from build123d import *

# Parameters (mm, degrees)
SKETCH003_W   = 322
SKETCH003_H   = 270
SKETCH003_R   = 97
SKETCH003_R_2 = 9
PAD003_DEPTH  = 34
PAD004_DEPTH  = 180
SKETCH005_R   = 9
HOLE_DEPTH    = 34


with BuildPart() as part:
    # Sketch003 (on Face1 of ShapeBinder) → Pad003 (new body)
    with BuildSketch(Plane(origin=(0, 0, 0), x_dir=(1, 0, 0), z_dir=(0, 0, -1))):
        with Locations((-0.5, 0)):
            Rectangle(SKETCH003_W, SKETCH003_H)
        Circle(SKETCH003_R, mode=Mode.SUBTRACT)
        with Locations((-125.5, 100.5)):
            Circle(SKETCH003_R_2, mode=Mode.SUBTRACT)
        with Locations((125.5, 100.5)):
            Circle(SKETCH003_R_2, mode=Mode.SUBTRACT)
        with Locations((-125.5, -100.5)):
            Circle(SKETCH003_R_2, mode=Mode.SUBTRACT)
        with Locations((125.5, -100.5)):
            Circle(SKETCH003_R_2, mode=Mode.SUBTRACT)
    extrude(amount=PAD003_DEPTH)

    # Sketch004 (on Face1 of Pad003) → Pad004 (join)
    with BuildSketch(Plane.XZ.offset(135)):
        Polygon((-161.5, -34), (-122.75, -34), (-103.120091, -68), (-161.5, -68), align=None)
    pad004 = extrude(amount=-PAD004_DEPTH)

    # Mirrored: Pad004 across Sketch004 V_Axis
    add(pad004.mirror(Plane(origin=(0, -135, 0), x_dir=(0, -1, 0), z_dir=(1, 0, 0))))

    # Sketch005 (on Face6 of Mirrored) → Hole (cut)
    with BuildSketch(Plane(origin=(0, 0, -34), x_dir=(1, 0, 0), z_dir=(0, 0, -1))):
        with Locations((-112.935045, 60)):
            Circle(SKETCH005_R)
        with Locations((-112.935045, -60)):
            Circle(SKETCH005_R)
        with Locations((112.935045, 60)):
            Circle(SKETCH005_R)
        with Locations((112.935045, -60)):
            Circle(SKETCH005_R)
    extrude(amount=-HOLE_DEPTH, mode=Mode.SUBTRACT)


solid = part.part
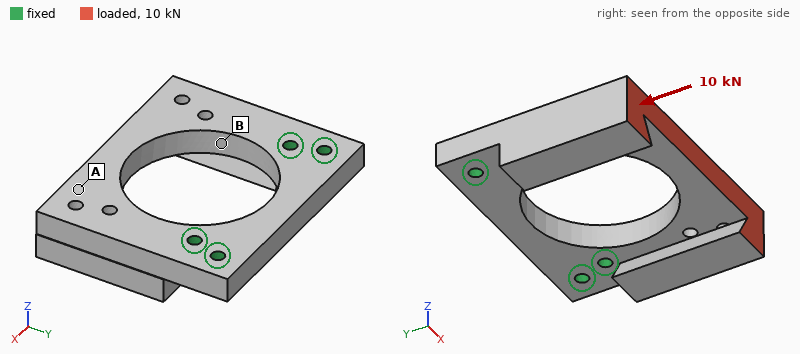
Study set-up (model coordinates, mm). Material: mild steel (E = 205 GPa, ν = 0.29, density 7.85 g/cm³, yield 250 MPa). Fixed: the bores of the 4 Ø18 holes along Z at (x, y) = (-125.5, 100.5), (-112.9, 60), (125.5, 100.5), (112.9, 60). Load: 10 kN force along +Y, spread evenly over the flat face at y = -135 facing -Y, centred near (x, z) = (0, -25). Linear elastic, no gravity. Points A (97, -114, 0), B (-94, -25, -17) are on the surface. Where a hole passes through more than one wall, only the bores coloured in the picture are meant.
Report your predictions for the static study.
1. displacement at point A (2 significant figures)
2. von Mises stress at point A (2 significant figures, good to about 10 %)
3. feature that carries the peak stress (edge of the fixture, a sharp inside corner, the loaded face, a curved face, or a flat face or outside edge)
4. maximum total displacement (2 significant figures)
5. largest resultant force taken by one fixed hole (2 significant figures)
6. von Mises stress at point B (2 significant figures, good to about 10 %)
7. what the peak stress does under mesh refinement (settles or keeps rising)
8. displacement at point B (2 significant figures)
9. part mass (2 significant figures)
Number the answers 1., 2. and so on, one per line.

1. 4.6 µm
2. 1.1 MPa
3. edge of the fixture
4. 6.8 µm
5. 3.8 kN
6. 5.2 MPa
7. keeps rising
8. 2.3 µm
9. 19 kg
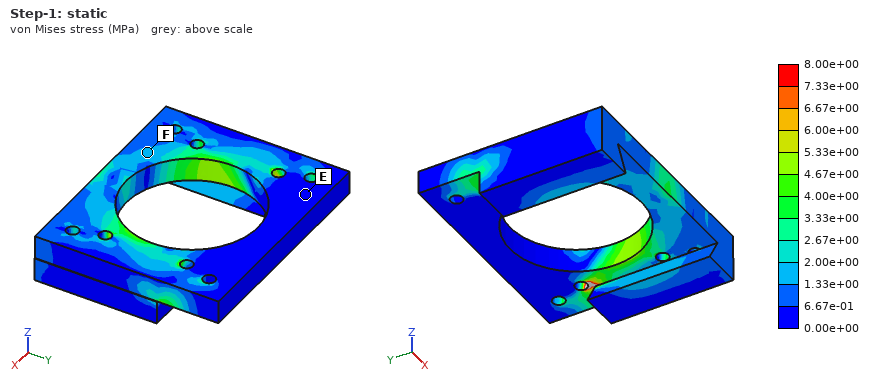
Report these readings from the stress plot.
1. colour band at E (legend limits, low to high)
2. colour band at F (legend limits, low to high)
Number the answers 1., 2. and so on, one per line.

1. 0.00e+00 to 6.67e-01 MPa
2. 1.33e+00 to 2.00e+00 MPa
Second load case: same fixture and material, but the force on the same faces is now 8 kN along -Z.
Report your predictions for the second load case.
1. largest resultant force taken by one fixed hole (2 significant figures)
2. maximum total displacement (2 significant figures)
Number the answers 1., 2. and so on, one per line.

1. 9.4 kN
2. 0.13 mm
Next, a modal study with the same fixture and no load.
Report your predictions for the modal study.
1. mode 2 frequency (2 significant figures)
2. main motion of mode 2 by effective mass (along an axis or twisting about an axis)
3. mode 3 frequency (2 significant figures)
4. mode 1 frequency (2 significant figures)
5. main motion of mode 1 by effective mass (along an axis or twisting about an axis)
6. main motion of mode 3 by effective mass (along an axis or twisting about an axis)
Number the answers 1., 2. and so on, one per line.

1. 790 Hz
2. twisting about Y
3. 1200 Hz
4. 550 Hz
5. along Z
6. along X
